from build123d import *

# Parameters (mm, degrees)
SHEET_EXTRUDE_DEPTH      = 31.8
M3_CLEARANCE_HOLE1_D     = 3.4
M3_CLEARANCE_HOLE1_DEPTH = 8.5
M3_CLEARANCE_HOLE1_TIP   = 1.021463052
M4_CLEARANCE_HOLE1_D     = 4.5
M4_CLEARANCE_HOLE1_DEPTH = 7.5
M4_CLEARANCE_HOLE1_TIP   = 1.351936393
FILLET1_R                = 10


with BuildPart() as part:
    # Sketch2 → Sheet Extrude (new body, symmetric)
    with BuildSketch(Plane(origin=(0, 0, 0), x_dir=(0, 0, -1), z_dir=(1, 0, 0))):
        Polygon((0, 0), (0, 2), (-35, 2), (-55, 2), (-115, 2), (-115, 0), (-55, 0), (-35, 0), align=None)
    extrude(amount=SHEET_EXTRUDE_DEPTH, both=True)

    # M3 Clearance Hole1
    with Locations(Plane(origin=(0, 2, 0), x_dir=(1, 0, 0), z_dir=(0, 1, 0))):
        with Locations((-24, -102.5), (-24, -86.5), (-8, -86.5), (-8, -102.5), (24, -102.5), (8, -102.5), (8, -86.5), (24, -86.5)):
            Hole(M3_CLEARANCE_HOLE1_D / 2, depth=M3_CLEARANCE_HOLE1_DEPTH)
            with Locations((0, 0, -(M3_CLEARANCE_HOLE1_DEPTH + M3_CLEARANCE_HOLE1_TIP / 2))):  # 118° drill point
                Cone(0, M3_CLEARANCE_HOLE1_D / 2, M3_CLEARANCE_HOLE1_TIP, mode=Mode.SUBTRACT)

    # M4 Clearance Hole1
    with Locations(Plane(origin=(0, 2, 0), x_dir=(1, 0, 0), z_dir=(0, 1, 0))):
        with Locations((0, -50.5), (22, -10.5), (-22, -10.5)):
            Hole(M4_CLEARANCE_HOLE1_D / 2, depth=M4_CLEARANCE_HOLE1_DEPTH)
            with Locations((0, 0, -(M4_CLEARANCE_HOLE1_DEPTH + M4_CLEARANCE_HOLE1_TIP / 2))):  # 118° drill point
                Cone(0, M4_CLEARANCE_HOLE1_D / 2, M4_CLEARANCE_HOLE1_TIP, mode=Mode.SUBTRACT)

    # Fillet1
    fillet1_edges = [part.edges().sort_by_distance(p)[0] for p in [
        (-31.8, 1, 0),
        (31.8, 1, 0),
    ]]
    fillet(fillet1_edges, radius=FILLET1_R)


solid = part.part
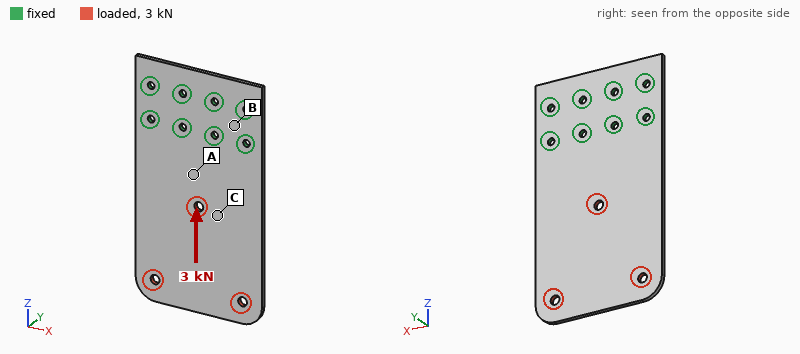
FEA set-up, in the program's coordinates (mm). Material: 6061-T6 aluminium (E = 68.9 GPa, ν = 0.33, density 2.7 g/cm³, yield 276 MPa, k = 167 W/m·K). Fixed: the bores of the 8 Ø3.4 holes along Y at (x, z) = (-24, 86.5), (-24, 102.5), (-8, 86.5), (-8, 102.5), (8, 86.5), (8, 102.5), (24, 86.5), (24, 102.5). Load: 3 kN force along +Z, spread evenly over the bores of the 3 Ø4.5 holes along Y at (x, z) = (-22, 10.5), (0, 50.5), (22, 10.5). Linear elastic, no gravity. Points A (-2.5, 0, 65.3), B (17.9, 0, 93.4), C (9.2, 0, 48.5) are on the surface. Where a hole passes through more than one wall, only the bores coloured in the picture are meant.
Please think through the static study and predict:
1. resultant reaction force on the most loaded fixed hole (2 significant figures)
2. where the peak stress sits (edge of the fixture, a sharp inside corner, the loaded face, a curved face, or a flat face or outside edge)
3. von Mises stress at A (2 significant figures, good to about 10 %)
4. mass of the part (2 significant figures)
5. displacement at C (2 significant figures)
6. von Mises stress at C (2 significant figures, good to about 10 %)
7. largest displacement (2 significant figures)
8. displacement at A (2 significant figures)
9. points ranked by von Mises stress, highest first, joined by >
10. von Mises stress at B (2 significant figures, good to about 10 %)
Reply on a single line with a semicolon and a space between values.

670 N; the loaded face; 29 MPa; 39 g; 14 µm; 19 MPa; 27 µm; 8.4 µm; A > C > B; 6.1 MPa
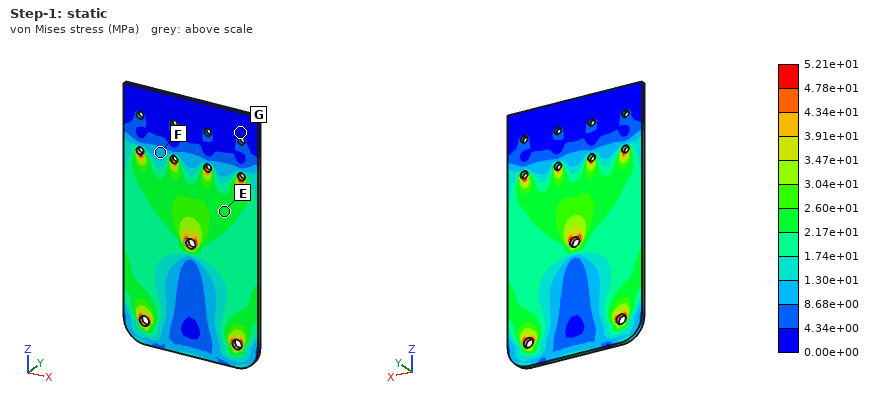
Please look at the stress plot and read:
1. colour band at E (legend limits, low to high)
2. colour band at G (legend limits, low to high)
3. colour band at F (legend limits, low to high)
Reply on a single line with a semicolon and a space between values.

2.17e+01 to 2.60e+01 MPa; 0.00e+00 to 4.34e+00 MPa; 8.68e+00 to 1.30e+01 MPa
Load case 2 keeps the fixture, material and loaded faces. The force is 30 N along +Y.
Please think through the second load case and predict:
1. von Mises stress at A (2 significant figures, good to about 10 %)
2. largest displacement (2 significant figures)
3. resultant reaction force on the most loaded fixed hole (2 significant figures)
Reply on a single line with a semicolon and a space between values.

26 MPa; 1.3 mm; 21 N
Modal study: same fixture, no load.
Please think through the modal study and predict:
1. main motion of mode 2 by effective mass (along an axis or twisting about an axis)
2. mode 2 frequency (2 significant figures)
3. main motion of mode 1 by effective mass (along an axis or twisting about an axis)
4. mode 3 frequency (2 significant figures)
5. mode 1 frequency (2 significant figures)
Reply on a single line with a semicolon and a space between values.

twisting about Z; 710 Hz; along Y; 1400 Hz; 230 Hz
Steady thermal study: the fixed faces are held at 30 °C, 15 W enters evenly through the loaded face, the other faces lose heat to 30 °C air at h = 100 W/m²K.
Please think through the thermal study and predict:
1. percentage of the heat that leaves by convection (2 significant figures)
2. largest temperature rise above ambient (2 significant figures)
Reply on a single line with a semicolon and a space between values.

70 %; 21 K
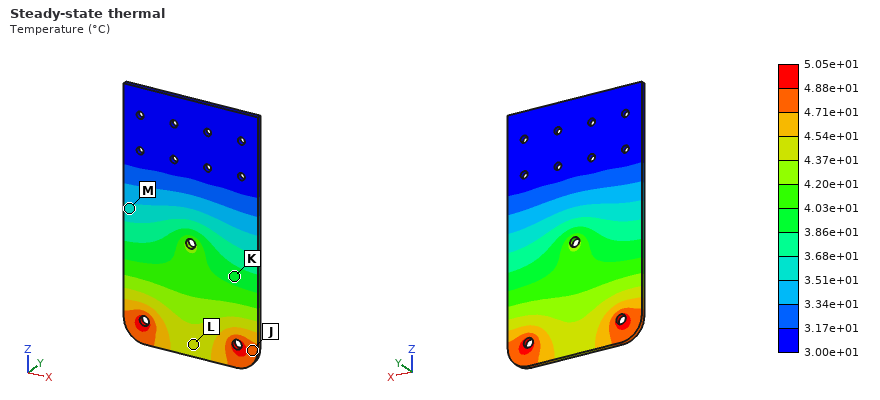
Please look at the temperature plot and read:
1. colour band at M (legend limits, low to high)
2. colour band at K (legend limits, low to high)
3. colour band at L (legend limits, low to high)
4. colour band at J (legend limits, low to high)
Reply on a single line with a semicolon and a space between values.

3.51e+01 to 3.68e+01 °C; 3.86e+01 to 4.03e+01 °C; 4.37e+01 to 4.54e+01 °C; 4.71e+01 to 4.88e+01 °C
